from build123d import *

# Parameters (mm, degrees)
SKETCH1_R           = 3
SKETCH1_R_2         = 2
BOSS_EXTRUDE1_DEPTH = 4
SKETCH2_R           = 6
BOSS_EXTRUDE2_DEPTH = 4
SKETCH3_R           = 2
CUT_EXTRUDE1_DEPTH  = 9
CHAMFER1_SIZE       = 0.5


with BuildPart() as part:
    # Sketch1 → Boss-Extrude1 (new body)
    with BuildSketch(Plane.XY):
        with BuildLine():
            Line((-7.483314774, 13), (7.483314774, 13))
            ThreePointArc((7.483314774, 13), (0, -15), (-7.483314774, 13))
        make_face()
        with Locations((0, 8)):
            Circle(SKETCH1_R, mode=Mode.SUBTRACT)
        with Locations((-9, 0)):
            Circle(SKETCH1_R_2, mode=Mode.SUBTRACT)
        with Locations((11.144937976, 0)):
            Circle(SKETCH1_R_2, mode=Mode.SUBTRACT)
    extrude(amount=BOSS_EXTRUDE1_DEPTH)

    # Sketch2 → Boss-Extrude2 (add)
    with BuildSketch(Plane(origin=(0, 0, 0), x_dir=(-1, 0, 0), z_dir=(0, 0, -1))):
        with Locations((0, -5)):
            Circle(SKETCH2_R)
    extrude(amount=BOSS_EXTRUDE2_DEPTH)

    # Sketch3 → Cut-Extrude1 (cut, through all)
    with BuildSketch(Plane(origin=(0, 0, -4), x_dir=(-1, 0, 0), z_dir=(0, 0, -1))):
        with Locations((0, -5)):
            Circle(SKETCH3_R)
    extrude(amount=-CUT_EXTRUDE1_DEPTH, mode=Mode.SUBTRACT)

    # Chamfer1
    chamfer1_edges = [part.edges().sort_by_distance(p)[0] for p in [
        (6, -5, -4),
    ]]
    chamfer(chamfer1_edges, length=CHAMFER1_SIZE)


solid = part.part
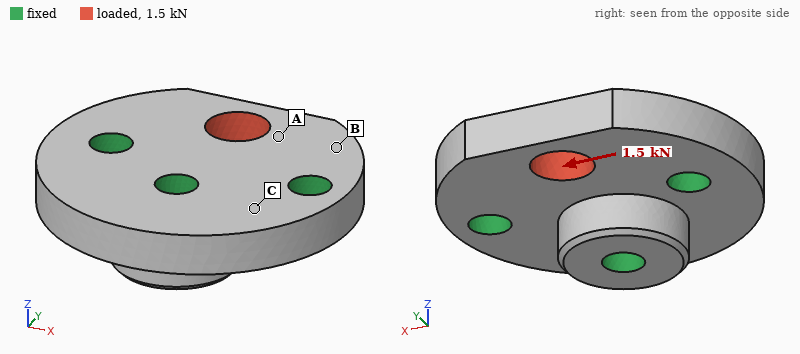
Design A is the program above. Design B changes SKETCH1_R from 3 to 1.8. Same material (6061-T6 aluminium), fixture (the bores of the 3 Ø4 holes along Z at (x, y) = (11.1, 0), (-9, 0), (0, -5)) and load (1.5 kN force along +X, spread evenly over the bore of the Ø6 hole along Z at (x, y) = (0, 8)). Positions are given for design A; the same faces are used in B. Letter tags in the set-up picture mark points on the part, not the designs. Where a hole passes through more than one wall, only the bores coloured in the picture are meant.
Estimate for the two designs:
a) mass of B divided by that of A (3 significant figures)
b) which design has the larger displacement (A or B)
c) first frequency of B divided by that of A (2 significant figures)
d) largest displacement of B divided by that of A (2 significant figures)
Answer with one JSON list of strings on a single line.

["1.03", "A", "0.98", "0.82"]
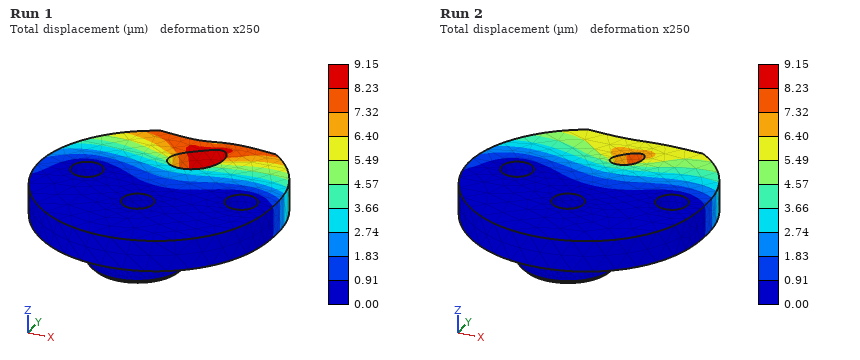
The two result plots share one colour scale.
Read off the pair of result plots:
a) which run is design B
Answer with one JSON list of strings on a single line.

["Run 2"]
